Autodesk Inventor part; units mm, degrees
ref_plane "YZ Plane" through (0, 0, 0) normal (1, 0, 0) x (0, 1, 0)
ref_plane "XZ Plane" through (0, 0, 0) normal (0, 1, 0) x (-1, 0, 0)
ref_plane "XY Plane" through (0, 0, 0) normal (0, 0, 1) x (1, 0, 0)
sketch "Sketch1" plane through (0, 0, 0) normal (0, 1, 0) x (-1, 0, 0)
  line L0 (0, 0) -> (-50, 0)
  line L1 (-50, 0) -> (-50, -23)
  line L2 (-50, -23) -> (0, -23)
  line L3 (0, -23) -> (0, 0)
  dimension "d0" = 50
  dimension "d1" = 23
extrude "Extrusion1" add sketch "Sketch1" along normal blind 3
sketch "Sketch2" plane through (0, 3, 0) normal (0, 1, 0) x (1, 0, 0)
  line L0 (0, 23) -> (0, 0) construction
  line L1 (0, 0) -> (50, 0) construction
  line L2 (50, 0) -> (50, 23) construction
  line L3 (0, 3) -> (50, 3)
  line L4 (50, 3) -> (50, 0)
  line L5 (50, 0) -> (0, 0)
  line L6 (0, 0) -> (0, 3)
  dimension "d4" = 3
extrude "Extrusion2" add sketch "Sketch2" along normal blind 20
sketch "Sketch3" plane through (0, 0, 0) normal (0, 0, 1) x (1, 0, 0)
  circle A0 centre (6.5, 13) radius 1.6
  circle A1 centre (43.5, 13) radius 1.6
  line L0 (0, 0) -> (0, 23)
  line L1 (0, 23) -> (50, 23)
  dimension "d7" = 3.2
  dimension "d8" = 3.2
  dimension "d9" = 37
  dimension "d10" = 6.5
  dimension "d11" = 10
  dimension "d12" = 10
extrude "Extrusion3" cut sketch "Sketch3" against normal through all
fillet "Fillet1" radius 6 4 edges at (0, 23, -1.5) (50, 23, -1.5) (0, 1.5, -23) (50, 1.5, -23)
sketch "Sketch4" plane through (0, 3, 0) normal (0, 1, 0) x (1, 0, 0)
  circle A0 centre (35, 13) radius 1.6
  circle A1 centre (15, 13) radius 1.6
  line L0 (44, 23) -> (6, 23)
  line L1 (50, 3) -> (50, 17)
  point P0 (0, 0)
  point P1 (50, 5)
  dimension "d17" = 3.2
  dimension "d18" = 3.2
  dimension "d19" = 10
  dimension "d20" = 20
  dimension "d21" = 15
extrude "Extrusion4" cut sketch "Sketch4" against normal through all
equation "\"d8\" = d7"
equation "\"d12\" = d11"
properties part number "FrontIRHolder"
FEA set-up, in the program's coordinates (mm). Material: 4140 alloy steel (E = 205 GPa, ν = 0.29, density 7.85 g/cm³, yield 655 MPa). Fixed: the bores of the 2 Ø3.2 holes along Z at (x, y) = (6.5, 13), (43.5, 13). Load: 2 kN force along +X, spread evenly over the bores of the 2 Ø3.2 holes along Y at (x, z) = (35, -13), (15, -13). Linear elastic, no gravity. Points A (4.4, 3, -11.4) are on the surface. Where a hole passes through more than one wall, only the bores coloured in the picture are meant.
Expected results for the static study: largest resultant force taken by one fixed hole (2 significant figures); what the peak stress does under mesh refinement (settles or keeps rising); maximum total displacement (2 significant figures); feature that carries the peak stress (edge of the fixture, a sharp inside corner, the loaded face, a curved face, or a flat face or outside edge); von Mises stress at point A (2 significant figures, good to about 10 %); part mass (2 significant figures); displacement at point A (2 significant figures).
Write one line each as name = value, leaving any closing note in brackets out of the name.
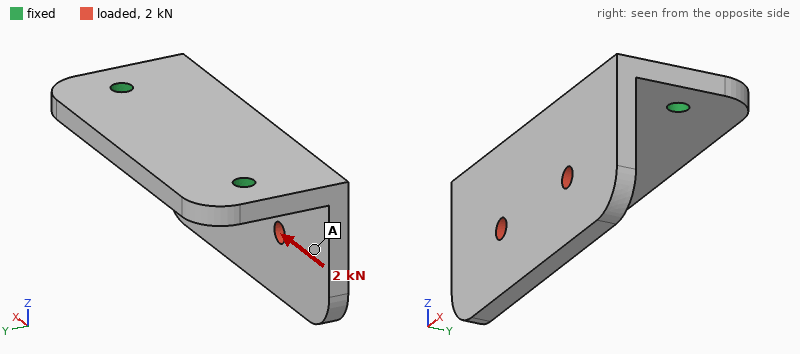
largest resultant force taken by one fixed hole = 1.3 kN
what the peak stress does under mesh refinement = keeps rising
maximum total displacement = 54 µm
feature that carries the peak stress = edge of the fixture
von Mises stress at point A = 43 MPa
part mass = 49 g
displacement at point A = 35 µm
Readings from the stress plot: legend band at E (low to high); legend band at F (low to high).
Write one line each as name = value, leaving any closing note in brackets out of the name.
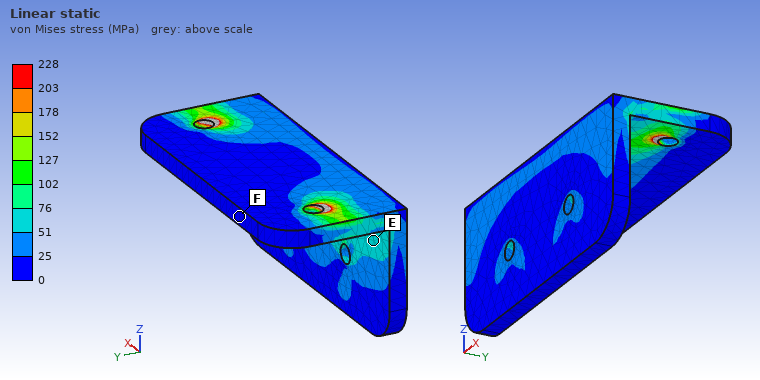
legend band at E = 51 to 76 MPa
legend band at F = 0 to 25 MPa
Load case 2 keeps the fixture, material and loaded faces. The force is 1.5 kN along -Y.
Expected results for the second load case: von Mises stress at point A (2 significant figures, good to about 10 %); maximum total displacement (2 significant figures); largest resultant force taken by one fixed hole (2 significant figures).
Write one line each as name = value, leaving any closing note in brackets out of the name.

von Mises stress at point A = 53 MPa
maximum total displacement = 0.28 mm
largest resultant force taken by one fixed hole = 770 N
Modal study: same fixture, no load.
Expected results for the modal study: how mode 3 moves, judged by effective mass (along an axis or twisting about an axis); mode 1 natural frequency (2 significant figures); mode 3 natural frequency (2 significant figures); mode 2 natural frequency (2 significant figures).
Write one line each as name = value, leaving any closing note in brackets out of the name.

how mode 3 moves, judged by effective mass = along Z
mode 1 natural frequency = 2800 Hz
mode 3 natural frequency = 7900 Hz
mode 2 natural frequency = 5200 Hz
